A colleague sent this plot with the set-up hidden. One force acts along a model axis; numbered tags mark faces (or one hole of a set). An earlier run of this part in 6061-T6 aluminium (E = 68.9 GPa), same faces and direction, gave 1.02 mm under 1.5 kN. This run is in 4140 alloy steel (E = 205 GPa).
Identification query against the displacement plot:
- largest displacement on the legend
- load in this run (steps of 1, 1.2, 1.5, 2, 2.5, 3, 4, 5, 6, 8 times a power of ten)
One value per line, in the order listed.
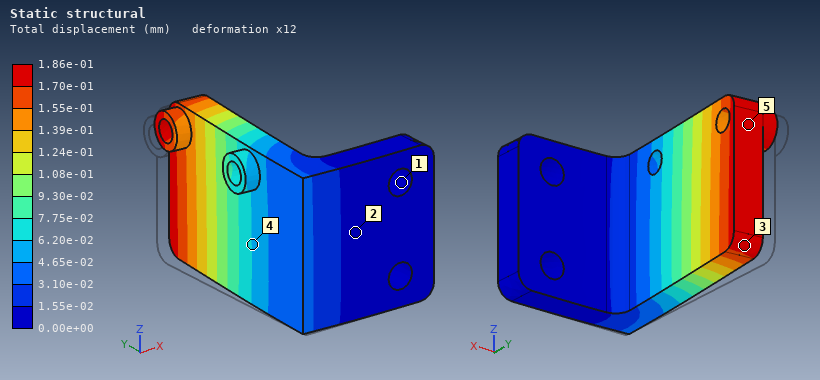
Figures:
1.86e-01 mm
800 N
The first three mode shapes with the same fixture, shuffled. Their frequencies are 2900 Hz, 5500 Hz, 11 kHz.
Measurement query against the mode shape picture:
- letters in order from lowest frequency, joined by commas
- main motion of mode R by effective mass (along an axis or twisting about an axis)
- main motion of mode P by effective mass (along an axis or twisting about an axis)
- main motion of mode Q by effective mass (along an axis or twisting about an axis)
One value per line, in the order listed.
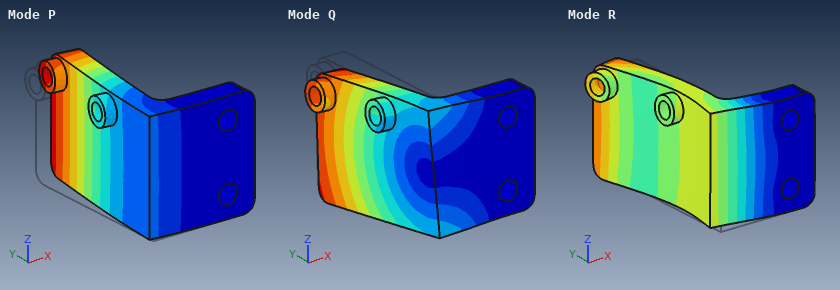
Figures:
P, Q, R
along Y
along X
along Z
